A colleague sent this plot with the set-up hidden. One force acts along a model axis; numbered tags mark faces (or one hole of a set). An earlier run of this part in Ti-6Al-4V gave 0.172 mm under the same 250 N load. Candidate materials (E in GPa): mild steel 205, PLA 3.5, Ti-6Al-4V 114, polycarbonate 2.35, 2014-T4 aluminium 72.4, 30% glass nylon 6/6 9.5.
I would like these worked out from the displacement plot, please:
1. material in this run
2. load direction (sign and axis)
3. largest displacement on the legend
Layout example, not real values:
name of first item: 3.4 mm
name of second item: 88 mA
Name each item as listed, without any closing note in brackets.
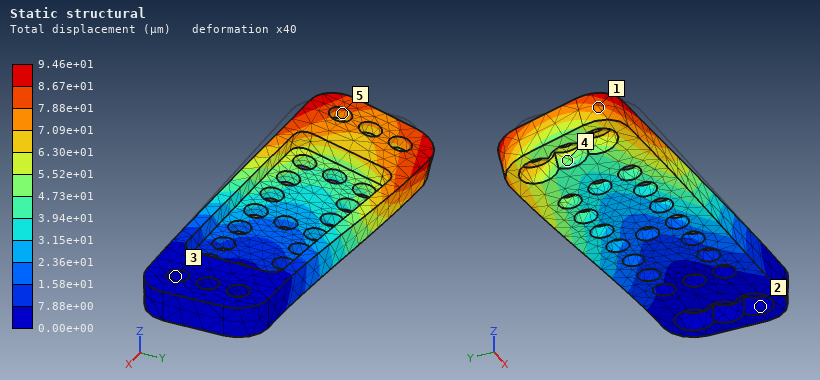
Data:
material in this run: mild steel
load direction: +Y
largest displacement on the legend: 9.46e+01 µm
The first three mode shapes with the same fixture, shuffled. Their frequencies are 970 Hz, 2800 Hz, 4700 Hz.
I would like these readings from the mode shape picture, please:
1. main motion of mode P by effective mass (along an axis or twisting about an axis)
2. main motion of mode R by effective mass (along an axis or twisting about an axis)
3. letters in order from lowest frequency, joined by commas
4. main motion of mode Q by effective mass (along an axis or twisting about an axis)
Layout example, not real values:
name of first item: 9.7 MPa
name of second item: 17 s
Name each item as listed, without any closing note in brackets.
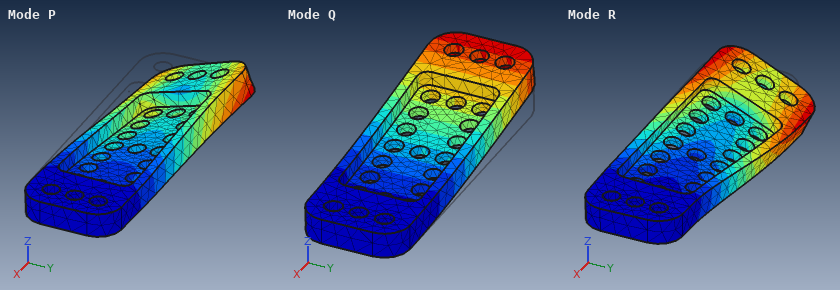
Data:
main motion of mode P by effective mass: along Y
main motion of mode R by effective mass: along Y
letters in order from lowest frequency, joined by commas: Q, R, P
main motion of mode Q by effective mass: along Z
